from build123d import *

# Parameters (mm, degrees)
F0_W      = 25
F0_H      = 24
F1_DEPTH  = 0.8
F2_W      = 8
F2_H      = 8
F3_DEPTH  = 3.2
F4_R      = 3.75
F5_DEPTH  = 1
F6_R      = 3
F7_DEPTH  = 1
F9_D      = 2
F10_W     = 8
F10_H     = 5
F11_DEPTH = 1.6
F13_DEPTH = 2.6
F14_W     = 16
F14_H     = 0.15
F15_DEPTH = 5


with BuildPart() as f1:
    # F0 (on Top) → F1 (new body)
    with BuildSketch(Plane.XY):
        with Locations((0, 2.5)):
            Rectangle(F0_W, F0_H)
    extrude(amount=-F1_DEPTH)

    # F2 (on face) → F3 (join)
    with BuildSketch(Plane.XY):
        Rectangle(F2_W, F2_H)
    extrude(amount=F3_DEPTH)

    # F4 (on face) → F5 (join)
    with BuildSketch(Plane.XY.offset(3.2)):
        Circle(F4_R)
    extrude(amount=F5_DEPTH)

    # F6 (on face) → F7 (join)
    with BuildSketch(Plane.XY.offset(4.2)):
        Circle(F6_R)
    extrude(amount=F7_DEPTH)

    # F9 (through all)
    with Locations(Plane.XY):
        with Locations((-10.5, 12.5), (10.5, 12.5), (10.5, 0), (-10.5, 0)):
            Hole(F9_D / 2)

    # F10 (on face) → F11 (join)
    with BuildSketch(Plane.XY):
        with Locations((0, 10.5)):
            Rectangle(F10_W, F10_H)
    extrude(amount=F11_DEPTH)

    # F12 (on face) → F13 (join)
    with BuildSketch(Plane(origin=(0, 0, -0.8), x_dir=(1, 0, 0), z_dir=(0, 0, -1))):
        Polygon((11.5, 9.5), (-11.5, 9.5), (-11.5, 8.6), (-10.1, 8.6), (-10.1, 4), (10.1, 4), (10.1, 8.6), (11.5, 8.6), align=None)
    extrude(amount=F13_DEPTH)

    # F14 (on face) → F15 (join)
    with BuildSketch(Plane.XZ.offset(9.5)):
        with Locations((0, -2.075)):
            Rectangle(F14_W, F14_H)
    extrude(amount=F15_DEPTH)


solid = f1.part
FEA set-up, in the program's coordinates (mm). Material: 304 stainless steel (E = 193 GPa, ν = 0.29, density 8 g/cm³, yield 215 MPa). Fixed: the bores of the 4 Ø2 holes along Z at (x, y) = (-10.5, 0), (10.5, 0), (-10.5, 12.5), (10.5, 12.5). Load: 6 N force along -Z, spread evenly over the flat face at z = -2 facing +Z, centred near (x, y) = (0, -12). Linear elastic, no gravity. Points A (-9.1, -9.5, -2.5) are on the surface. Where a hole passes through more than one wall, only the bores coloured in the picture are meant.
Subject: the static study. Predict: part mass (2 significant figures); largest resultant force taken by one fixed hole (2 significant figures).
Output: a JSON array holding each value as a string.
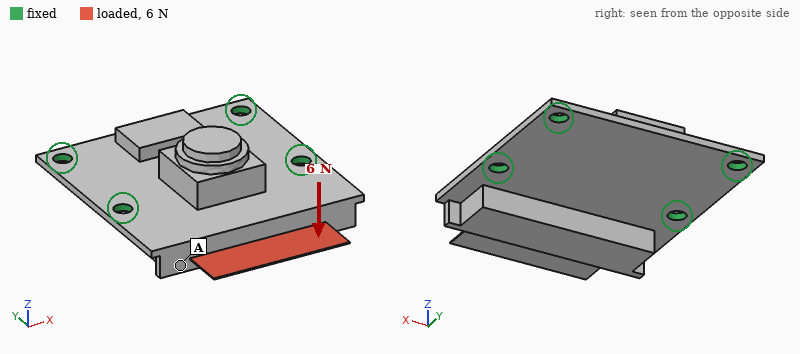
["8.9 g", "4.5 N"]
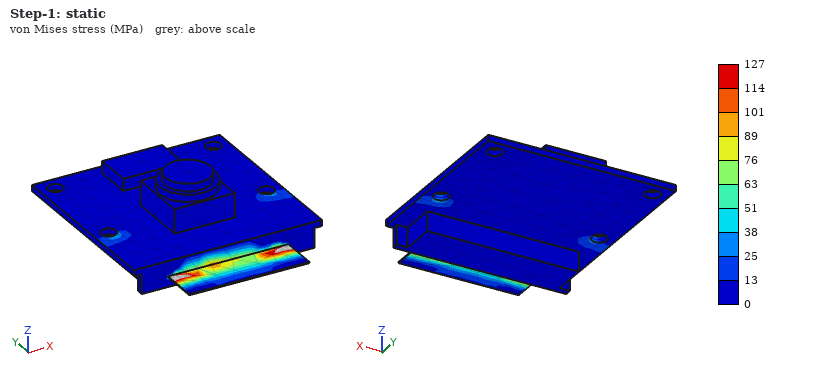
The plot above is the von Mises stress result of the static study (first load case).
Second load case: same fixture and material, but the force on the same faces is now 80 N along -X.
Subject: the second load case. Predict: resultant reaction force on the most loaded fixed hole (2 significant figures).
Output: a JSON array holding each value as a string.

["57 N"]
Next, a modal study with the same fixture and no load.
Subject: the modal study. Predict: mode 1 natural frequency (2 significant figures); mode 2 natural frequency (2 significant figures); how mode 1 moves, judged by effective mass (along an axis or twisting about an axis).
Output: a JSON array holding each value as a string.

["4000 Hz", "5300 Hz", "along Z"]
